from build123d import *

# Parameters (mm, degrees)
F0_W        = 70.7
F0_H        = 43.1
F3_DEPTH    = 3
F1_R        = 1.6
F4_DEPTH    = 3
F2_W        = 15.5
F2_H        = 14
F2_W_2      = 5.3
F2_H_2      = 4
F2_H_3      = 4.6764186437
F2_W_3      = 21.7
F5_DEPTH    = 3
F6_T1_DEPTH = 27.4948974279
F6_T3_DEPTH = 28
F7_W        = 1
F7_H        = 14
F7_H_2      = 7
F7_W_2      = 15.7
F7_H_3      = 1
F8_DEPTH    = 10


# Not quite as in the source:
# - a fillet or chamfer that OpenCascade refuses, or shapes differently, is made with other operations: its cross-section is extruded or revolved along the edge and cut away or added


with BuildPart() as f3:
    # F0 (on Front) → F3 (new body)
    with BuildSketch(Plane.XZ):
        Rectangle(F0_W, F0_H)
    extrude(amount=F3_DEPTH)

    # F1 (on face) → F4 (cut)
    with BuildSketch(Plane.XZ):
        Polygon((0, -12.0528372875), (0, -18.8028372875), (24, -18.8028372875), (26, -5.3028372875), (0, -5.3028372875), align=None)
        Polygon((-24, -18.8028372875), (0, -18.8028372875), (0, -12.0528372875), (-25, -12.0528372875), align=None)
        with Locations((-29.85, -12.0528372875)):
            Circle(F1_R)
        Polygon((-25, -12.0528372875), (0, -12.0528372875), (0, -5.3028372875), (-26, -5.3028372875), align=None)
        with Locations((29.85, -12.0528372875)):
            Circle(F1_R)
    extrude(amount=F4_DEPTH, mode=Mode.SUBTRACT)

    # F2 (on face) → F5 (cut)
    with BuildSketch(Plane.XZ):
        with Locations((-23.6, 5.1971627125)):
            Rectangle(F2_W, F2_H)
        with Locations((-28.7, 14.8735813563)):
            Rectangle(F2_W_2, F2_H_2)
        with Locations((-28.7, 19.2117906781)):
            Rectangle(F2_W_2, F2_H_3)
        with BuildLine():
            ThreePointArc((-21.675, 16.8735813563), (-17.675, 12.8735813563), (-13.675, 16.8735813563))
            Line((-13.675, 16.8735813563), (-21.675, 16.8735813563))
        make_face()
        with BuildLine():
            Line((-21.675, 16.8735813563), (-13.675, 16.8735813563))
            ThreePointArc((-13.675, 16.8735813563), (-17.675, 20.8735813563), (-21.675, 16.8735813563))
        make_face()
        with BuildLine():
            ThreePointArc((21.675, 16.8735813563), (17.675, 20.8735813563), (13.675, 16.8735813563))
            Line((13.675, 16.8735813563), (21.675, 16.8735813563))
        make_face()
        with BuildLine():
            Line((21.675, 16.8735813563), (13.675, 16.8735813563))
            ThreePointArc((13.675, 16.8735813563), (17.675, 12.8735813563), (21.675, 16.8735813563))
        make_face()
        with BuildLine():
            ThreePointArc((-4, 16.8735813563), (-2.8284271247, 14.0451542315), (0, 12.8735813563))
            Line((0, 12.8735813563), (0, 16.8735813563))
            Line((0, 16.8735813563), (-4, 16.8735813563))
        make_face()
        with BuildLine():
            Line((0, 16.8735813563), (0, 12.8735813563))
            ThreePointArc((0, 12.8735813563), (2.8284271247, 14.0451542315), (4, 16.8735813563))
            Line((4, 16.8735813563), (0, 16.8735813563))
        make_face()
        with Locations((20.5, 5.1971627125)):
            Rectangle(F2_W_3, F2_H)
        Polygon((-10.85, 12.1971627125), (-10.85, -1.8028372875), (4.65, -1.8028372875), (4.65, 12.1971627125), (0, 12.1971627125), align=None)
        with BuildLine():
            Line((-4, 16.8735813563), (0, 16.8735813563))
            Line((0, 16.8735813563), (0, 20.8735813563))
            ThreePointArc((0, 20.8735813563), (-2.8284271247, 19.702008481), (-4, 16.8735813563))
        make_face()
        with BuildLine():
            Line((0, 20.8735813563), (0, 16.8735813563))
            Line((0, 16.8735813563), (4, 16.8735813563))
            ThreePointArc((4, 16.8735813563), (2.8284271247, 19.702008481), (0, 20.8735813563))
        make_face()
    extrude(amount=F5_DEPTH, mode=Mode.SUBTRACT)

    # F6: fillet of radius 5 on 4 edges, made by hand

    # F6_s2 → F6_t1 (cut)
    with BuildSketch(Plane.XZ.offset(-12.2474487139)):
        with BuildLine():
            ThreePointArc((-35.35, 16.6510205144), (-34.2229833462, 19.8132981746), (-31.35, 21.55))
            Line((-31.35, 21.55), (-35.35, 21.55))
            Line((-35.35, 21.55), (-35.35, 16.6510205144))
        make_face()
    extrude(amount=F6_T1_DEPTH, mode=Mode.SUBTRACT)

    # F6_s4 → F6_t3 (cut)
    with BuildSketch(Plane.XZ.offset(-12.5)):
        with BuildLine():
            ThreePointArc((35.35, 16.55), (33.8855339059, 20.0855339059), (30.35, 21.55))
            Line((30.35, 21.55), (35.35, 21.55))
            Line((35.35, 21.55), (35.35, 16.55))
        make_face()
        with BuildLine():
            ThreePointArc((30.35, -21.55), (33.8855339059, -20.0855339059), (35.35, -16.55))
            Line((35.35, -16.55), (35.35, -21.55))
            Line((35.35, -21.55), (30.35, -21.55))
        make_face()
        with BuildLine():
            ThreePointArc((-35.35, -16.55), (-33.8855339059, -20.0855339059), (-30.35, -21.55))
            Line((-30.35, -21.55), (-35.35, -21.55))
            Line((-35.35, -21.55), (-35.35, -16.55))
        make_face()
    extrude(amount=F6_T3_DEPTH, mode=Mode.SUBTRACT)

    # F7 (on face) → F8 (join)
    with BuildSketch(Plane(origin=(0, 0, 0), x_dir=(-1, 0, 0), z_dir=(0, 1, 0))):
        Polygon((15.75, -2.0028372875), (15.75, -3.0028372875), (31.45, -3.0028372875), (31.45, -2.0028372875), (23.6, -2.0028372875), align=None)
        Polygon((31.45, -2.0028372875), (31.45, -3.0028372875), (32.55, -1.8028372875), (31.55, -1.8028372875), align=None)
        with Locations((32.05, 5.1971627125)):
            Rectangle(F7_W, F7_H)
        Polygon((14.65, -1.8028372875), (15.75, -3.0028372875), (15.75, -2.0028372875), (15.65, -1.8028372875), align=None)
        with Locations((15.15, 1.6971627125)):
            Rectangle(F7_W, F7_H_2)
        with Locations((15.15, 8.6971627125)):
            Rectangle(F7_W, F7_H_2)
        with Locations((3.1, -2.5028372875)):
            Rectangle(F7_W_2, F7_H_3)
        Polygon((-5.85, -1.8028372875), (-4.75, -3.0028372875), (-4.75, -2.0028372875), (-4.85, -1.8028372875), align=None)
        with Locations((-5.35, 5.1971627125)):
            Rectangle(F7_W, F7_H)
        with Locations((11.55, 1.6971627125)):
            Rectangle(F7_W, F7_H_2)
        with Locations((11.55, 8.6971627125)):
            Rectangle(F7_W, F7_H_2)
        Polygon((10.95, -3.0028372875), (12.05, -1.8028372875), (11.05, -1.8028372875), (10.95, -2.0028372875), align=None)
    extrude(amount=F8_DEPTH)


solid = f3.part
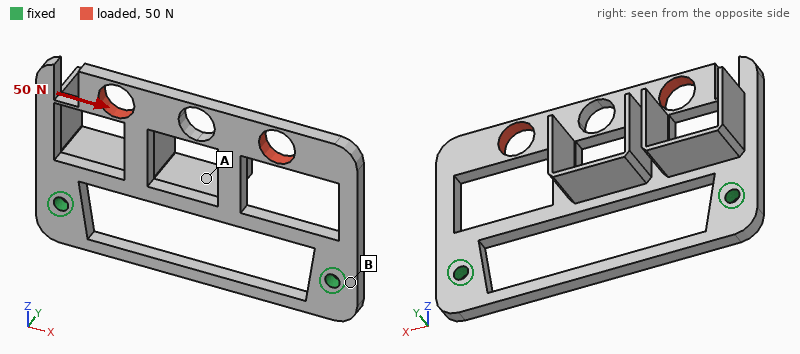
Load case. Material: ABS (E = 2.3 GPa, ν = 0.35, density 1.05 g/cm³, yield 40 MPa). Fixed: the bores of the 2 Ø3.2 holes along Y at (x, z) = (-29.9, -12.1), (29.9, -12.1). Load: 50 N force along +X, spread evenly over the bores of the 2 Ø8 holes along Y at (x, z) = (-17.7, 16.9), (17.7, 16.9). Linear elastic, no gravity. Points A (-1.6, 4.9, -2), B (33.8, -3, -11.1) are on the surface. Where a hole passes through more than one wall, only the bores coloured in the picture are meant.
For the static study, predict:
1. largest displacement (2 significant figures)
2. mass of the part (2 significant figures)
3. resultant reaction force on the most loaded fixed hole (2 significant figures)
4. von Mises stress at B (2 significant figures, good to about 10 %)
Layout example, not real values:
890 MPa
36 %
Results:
0.42 mm
5.4 g
32 N
2.7 MPa
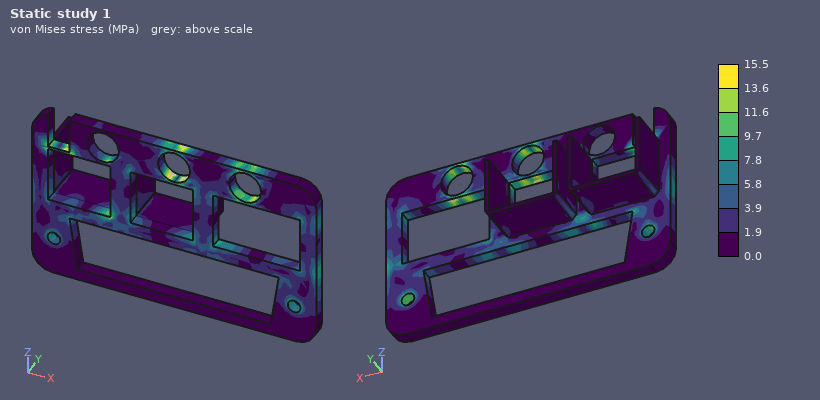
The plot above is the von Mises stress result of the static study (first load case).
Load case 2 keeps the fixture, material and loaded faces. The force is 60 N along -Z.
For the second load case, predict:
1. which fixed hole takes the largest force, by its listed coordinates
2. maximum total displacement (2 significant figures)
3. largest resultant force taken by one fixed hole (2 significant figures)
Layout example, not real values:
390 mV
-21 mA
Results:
(-29.9, -12.1)
0.47 mm
36 N
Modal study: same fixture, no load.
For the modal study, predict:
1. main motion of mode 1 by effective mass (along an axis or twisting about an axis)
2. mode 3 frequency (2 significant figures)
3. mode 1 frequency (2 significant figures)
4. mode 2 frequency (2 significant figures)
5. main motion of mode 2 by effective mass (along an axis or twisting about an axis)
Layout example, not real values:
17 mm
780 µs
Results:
along Y
960 Hz
340 Hz
740 Hz
twisting about Z
